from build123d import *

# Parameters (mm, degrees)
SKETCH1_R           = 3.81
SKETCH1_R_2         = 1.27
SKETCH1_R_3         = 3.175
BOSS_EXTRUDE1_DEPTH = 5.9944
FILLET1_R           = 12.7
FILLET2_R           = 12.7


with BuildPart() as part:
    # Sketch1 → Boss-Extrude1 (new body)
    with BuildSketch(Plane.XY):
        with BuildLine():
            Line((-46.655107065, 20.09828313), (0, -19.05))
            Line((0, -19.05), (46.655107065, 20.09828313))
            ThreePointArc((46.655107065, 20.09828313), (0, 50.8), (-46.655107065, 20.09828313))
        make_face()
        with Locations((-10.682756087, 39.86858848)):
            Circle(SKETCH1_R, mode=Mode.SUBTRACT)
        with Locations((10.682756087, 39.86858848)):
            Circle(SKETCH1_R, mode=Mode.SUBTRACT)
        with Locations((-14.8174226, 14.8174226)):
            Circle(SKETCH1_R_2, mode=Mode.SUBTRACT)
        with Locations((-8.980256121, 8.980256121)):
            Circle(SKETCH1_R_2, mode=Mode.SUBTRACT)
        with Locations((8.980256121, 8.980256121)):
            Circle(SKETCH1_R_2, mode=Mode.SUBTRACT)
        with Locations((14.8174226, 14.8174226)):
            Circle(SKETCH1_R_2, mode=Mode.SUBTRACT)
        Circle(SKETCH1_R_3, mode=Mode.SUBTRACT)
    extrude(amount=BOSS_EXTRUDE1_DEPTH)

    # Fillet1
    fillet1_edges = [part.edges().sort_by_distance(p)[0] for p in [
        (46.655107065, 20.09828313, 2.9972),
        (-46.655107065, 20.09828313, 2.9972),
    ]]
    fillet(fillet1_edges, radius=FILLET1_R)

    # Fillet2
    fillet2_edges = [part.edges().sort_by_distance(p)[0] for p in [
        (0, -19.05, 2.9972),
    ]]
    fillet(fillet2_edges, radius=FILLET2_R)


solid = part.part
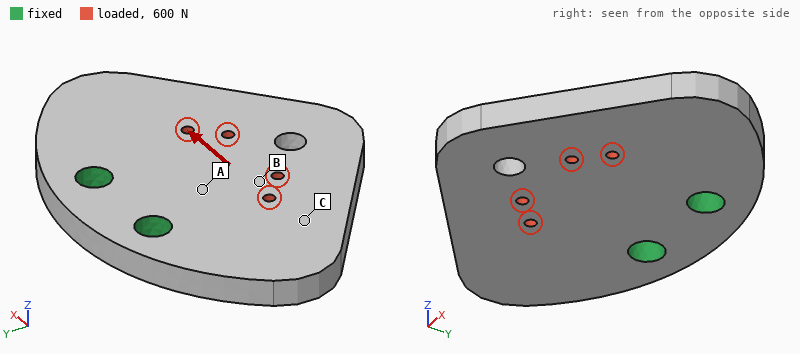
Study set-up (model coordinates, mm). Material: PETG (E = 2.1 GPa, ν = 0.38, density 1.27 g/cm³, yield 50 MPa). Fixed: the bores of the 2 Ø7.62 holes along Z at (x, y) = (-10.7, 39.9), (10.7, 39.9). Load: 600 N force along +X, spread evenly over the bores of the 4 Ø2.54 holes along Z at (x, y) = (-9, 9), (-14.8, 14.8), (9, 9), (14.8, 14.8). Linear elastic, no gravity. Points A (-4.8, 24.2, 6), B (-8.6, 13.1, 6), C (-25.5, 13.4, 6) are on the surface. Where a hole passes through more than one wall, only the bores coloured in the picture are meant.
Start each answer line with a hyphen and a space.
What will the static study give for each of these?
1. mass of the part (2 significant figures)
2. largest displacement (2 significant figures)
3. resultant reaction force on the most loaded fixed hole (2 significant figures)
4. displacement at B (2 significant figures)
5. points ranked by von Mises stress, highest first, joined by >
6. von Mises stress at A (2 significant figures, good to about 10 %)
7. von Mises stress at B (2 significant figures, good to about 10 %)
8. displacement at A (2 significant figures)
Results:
- 28 g
- 0.24 mm
- 630 N
- 0.14 mm
- A > B > C
- 5.6 MPa
- 3.3 MPa
- 0.075 mm
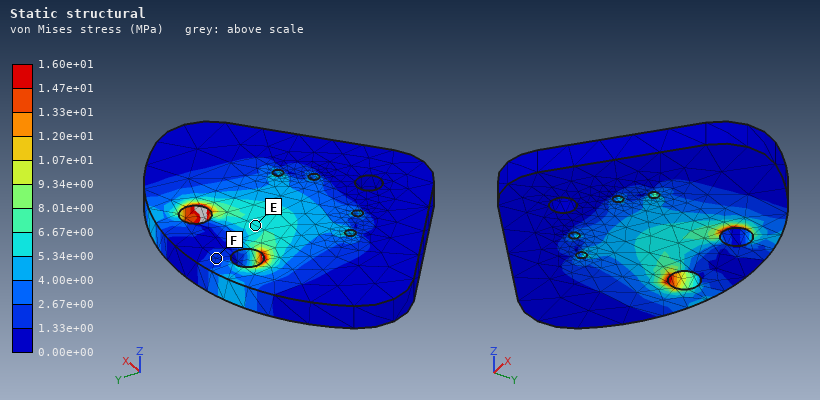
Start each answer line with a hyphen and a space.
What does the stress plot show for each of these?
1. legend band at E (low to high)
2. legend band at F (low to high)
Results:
- 5.34e+00 to 6.67e+00 MPa
- 1.33e+00 to 2.67e+00 MPa
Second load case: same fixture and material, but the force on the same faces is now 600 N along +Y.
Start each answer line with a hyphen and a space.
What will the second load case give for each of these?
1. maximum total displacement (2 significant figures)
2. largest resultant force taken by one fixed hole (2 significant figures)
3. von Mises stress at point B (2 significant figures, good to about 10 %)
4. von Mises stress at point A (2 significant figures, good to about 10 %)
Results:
- 37 µm
- 300 N
- 2.9 MPa
- 2.2 MPa
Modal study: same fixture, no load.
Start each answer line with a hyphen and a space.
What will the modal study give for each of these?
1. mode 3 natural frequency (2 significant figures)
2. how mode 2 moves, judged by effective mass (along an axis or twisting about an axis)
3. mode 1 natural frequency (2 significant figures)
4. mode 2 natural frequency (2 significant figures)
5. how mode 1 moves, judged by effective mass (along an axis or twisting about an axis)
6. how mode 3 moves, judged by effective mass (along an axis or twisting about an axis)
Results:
- 1400 Hz
- twisting about Y
- 600 Hz
- 960 Hz
- along Z
- along Z
